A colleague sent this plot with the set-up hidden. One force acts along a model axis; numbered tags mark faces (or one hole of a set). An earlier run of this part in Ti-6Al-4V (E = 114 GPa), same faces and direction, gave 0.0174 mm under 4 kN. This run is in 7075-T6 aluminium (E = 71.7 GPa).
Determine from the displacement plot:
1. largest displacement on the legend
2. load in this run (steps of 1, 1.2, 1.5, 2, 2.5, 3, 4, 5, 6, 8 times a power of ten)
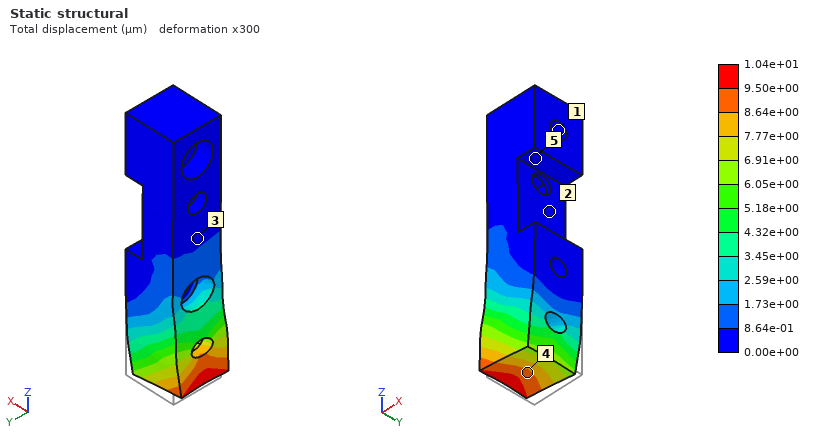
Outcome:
1.04e+01 µm
1.5 kN
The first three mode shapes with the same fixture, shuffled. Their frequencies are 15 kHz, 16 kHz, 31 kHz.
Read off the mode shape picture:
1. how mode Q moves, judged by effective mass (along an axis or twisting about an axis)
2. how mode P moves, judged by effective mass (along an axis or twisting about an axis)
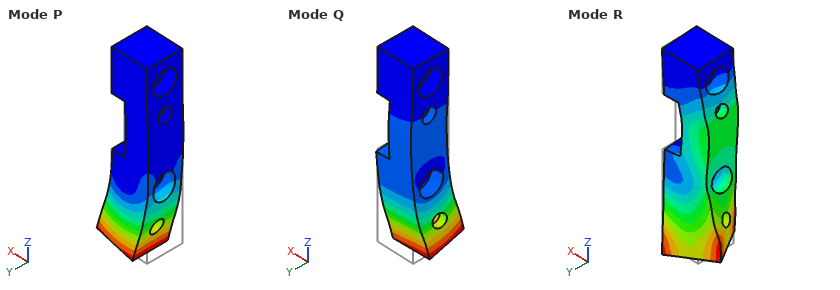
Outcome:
along Y
along X
